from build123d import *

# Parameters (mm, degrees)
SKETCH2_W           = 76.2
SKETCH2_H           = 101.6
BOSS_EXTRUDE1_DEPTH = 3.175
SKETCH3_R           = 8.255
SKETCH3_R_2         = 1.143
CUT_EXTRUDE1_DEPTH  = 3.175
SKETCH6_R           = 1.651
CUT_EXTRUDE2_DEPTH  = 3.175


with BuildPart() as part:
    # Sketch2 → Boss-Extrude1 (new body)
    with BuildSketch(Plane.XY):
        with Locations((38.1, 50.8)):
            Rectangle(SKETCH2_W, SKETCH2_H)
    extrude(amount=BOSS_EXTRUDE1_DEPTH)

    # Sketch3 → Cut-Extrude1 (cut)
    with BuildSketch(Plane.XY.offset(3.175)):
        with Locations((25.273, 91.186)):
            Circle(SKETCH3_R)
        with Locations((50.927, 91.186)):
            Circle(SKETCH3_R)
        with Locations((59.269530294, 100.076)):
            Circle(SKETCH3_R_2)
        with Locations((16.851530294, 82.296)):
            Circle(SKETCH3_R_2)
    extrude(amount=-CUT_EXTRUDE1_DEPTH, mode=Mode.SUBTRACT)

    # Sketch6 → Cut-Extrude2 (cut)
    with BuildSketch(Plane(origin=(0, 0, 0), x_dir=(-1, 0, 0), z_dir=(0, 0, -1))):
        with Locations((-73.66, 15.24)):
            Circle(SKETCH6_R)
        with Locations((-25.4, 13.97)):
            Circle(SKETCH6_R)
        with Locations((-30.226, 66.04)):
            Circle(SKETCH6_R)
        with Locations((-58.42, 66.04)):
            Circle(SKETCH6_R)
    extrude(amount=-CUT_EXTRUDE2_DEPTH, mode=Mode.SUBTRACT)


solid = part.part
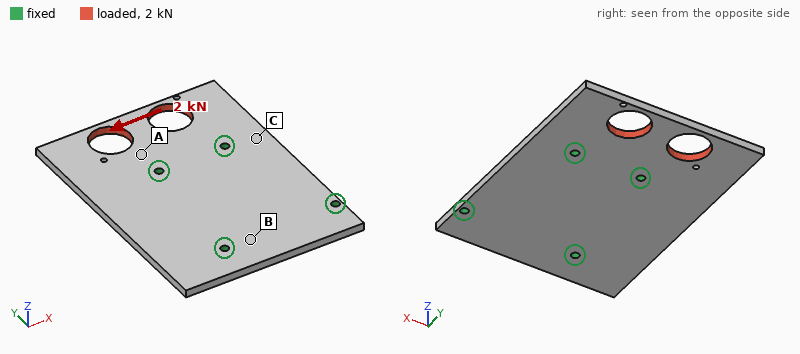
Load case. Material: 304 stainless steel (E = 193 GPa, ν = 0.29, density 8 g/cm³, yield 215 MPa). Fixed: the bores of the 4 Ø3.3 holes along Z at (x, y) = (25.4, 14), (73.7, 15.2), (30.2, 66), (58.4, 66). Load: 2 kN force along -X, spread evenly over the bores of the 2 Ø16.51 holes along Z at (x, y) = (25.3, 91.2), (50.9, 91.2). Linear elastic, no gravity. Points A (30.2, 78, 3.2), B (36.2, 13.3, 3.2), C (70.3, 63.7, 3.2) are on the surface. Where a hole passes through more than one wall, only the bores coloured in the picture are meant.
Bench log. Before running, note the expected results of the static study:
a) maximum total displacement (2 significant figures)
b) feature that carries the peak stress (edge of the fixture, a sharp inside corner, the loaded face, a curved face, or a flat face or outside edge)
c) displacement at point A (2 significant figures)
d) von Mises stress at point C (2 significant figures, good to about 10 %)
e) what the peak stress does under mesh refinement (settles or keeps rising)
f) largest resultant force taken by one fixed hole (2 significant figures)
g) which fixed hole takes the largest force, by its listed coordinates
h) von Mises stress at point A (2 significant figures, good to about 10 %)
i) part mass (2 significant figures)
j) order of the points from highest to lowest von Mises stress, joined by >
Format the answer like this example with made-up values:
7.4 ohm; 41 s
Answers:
13 µm; edge of the fixture; 3.2 µm; 14 MPa; keeps rising; 1.5 kN; (30.2, 66); 27 MPa; 180 g; A > C > B
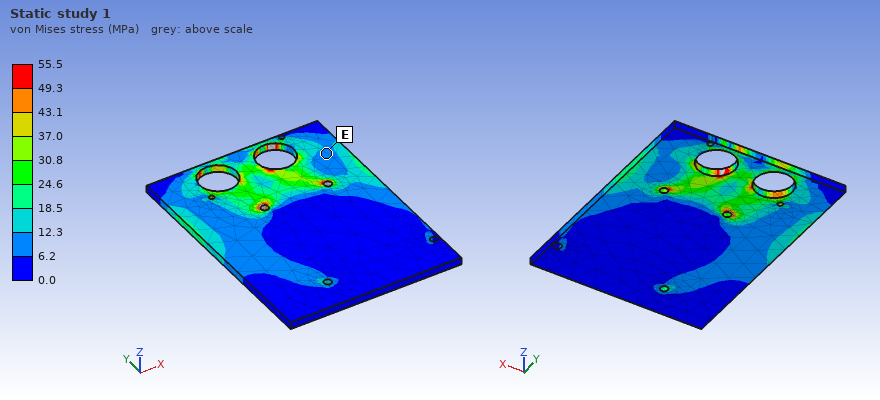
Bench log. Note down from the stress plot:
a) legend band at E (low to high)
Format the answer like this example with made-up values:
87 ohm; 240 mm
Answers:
6.2 to 12.3 MPa
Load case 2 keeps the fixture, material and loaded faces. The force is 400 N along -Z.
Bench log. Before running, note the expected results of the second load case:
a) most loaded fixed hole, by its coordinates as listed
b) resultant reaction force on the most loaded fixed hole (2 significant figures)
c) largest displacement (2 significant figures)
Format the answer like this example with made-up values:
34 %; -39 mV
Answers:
(30.2, 66); 310 N; 0.13 mm
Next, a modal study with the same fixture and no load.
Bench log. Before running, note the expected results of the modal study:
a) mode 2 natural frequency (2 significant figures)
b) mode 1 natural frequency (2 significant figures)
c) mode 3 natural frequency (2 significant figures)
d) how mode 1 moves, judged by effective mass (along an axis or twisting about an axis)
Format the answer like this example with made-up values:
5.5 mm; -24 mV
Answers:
2200 Hz; 1700 Hz; 2700 Hz; along Z
